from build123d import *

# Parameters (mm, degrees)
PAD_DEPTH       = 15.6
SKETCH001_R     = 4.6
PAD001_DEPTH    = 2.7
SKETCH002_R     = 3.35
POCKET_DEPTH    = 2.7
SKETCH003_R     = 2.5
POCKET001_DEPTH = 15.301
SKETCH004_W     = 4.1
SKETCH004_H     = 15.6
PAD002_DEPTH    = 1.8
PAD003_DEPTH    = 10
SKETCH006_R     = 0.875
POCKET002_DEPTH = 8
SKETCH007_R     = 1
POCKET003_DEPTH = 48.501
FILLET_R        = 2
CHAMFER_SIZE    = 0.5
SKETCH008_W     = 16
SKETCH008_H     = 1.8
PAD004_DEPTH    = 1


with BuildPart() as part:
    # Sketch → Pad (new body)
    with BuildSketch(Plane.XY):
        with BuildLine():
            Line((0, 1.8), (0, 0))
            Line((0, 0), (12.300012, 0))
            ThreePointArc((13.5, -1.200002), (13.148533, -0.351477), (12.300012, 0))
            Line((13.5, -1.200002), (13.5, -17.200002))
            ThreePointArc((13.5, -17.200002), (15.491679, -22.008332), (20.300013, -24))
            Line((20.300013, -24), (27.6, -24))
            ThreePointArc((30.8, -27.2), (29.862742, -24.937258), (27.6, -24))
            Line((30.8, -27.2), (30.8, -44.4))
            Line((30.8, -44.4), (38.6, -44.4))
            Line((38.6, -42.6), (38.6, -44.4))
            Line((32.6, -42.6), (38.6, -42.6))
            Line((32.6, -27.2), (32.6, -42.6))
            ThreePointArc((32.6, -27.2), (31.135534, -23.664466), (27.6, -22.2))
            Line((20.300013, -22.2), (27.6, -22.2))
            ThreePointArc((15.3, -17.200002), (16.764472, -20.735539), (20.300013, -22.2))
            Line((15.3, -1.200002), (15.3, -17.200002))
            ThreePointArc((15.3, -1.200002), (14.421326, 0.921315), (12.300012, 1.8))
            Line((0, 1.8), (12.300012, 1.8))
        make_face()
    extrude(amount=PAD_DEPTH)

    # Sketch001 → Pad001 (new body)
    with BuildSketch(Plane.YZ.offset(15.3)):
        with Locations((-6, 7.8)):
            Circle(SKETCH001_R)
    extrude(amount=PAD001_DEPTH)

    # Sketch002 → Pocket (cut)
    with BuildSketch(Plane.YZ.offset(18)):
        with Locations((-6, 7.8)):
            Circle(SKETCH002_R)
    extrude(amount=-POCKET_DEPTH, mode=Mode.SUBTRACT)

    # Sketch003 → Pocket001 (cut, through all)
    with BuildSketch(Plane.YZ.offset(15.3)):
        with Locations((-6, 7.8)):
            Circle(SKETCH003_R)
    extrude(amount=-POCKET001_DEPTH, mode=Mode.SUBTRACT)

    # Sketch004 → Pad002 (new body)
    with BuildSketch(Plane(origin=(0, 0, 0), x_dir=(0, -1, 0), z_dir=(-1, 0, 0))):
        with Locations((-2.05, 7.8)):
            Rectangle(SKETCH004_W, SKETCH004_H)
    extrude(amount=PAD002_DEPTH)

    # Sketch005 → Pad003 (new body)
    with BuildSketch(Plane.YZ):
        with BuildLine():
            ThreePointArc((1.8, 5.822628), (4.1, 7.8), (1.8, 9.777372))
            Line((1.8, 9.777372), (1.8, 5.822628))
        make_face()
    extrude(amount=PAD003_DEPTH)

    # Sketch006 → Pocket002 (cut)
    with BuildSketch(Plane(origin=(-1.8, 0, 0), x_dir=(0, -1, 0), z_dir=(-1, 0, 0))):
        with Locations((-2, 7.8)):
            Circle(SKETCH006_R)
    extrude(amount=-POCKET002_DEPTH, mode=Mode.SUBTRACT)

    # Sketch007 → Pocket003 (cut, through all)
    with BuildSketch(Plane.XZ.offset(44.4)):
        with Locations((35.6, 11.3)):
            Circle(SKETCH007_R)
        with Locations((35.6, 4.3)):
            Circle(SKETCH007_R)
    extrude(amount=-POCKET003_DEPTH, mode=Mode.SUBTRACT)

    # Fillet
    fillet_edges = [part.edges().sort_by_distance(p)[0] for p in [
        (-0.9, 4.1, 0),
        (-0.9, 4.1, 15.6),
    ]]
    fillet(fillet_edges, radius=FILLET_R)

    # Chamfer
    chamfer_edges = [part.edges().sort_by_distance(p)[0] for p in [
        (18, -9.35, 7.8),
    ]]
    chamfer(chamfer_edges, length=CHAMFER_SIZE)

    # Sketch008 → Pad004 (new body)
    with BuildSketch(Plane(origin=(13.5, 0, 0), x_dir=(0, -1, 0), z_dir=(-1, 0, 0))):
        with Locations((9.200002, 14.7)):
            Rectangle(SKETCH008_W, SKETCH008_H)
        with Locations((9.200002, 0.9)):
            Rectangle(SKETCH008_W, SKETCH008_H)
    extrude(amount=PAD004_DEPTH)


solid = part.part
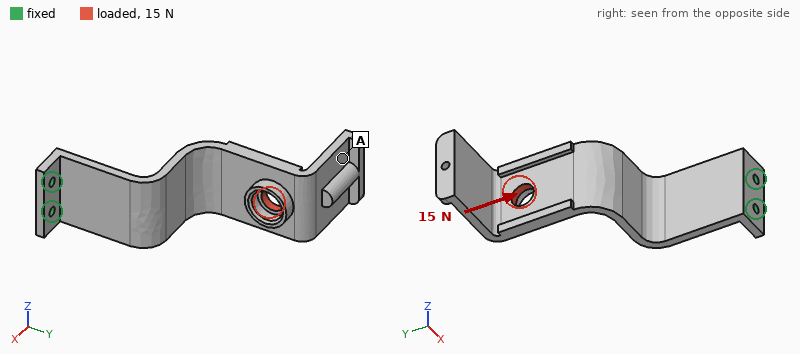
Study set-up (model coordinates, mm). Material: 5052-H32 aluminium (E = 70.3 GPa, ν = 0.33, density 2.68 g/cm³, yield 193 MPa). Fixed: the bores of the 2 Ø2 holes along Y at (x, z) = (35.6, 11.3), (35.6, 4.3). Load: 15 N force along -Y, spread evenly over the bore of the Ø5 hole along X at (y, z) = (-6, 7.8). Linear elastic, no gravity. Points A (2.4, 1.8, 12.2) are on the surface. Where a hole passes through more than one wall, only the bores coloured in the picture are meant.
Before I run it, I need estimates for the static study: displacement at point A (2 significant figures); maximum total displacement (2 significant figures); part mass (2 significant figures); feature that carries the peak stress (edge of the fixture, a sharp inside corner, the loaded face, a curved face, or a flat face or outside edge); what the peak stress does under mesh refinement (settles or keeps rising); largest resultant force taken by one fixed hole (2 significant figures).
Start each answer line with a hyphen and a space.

- 0.62 mm
- 0.69 mm
- 6.6 g
- edge of the fixture
- keeps rising
- 9.4 N
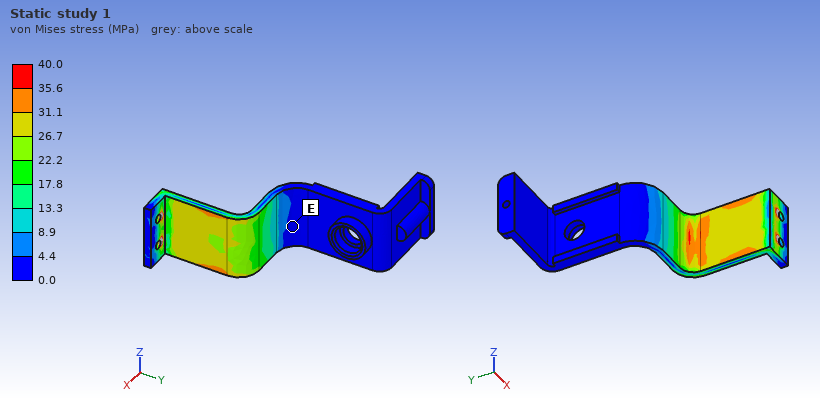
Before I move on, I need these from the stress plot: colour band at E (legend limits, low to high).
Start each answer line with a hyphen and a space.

- 0.0 to 4.4 MPa
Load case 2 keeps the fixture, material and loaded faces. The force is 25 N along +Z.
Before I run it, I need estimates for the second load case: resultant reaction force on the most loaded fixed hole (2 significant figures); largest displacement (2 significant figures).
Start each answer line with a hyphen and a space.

- 120 N
- 0.37 mm
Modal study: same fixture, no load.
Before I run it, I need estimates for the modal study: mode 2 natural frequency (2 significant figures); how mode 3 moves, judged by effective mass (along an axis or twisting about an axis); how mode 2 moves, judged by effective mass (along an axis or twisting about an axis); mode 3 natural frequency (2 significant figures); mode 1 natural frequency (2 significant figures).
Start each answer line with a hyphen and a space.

- 740 Hz
- along X
- along Z
- 2000 Hz
- 300 Hz
